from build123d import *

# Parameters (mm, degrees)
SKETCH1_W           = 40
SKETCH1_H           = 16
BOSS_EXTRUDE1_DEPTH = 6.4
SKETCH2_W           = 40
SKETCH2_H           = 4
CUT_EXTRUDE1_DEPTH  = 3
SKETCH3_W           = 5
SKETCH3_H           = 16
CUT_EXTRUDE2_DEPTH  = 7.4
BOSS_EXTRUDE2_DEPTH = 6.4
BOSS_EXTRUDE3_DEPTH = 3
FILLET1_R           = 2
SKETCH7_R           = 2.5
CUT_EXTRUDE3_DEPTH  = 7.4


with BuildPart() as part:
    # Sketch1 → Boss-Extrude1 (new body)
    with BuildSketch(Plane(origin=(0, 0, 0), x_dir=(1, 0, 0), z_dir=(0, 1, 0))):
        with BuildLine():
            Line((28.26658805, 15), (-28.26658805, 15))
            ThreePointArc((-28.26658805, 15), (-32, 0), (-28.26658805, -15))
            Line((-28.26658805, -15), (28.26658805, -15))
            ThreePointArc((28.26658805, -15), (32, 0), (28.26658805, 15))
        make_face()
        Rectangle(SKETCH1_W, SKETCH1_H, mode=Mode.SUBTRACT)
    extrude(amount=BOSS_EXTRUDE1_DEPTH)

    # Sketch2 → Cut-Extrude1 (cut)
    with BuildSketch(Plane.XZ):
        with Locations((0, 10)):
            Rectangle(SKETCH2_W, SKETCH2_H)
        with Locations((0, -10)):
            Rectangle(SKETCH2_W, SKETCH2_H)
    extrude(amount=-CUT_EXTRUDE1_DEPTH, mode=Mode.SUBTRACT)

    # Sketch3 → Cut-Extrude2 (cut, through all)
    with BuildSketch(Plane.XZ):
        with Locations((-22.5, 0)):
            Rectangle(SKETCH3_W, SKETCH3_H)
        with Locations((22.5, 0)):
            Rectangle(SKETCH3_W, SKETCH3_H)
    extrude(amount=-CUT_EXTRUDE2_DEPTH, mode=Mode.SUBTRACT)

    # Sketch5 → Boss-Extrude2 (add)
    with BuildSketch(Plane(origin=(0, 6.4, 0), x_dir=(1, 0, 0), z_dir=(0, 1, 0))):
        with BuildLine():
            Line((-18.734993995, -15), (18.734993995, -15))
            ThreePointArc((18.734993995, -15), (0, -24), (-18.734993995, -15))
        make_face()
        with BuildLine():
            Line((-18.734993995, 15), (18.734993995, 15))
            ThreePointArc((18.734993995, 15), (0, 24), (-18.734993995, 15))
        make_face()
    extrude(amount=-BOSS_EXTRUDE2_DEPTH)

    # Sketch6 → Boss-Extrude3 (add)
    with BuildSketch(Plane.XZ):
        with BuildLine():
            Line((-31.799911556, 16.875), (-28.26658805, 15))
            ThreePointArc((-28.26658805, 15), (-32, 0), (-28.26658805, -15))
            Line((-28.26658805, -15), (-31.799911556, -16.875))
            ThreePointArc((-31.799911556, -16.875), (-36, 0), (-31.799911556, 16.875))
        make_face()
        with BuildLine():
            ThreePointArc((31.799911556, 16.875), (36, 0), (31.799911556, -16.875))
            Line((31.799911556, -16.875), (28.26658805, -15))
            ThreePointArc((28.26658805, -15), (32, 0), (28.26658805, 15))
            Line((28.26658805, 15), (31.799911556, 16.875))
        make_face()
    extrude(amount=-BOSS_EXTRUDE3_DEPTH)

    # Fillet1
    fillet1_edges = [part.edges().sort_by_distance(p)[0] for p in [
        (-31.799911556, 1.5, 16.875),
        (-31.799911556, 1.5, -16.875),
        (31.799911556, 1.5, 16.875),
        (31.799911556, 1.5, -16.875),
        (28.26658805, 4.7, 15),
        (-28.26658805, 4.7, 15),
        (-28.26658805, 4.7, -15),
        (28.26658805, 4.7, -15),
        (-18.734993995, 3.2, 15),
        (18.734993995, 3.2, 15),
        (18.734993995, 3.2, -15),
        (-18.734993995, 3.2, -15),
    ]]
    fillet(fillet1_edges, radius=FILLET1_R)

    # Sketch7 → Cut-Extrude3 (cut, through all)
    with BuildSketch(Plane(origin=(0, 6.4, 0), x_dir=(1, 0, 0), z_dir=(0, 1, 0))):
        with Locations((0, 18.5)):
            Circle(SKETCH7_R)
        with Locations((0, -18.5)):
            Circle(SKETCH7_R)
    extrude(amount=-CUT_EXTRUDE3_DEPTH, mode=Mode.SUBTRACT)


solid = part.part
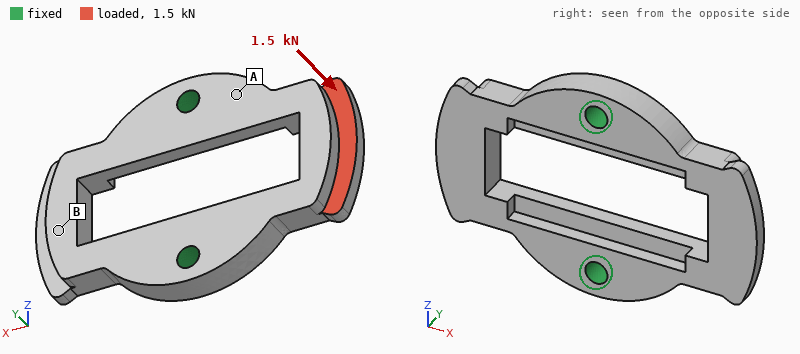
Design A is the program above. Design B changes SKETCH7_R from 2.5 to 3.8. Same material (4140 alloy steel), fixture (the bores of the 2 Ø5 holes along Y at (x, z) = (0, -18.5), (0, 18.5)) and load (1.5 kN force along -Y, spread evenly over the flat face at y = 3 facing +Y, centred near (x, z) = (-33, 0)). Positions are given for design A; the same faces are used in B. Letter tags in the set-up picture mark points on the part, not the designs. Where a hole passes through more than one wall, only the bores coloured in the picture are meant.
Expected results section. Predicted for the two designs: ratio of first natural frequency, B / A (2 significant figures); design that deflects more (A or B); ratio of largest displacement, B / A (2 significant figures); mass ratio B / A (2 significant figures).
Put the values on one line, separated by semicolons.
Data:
1.1; A; 0.90; 0.96
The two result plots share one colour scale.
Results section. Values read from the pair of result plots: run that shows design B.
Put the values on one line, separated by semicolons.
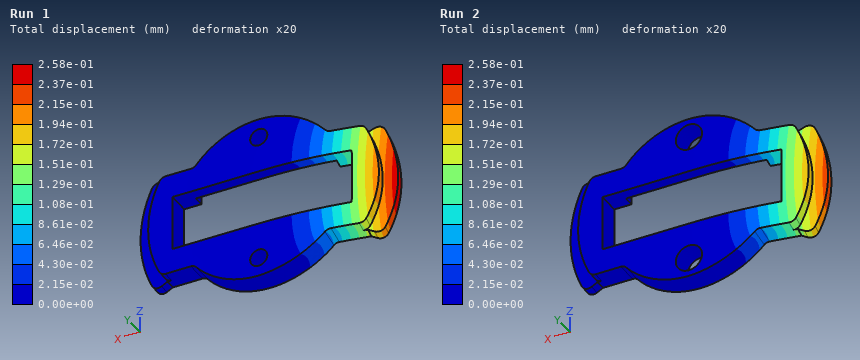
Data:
Run 2
